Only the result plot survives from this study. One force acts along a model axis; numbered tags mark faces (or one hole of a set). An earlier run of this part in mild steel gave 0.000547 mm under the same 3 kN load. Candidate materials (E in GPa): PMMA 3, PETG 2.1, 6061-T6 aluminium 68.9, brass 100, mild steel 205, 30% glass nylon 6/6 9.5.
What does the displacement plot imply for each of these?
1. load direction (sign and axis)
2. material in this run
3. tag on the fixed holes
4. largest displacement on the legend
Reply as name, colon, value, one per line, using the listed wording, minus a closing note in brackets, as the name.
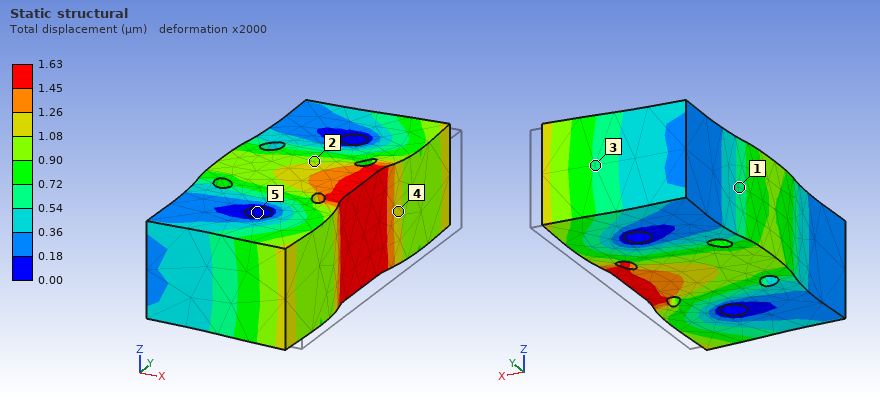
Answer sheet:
load direction: -X
material in this run: 6061-T6 aluminium
tag on the fixed holes: 5
largest displacement on the legend: 1.63 µm
